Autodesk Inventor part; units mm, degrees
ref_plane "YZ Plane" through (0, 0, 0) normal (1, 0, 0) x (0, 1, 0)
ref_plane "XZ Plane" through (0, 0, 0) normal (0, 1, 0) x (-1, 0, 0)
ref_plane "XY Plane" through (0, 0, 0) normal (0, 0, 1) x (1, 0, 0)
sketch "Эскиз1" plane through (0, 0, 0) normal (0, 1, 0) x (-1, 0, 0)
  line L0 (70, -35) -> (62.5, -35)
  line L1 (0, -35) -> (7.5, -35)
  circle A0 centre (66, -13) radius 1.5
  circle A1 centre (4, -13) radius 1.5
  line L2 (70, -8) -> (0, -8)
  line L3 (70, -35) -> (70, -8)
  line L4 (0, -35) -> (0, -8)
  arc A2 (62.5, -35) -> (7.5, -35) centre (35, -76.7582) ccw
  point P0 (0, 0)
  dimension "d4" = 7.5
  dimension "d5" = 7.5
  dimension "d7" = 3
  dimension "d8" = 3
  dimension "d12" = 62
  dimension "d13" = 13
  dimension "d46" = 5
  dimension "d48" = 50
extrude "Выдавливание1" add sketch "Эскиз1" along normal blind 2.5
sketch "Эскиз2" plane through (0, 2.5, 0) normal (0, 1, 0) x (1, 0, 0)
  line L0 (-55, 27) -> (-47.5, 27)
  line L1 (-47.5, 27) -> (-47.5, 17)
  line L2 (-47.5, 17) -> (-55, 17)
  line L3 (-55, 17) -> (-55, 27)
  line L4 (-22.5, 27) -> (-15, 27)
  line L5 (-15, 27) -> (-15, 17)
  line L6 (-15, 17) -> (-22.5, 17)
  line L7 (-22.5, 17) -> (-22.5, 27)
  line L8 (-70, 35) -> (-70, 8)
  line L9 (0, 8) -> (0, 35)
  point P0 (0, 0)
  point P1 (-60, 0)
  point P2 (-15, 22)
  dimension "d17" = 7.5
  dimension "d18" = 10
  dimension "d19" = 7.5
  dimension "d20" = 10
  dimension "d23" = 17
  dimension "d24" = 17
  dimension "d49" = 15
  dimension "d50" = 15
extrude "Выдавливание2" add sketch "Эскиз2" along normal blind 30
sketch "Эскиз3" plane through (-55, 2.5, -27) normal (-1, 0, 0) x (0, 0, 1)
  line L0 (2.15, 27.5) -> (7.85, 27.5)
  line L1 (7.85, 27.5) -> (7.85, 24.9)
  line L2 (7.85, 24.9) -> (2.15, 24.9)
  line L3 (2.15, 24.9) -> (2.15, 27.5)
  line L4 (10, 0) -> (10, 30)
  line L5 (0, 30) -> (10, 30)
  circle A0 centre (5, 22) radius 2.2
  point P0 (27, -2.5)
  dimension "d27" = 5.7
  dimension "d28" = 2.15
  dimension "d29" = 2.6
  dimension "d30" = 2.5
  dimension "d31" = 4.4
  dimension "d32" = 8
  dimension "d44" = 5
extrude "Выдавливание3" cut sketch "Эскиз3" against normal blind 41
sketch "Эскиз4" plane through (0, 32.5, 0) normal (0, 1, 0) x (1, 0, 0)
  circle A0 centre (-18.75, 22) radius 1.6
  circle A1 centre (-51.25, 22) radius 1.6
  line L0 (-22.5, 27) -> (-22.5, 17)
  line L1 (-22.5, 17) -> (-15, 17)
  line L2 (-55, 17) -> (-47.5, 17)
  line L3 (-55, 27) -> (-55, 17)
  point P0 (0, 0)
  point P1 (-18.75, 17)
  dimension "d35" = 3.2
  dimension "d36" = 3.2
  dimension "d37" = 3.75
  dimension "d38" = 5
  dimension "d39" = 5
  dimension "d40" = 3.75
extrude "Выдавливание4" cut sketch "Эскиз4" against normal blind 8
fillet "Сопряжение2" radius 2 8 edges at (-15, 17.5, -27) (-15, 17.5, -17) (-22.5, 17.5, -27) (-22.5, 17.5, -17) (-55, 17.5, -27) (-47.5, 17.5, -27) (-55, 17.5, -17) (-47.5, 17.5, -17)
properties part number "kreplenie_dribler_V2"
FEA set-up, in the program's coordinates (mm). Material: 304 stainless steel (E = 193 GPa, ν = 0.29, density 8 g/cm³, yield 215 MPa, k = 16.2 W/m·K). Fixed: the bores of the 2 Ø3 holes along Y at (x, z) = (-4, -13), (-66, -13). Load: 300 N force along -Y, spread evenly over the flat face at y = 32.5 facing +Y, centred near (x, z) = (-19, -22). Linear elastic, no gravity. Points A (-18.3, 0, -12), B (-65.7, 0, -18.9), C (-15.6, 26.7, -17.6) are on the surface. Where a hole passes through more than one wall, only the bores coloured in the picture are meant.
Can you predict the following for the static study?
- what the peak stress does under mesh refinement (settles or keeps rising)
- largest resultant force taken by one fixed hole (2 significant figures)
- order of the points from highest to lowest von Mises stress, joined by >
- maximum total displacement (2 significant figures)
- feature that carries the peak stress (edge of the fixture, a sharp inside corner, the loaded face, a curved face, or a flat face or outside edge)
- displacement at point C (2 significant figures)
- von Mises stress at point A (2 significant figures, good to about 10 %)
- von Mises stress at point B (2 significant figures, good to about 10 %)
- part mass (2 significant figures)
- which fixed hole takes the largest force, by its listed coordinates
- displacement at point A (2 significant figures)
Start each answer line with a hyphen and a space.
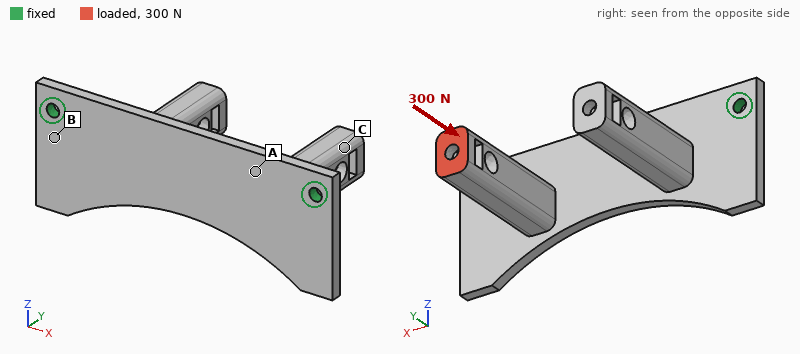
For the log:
- keeps rising
- 250 N
- B > A > C
- 0.14 mm
- edge of the fixture
- 0.10 mm
- 26 MPa
- 48 MPa
- 62 g
- (-4, -13)
- 0.024 mm
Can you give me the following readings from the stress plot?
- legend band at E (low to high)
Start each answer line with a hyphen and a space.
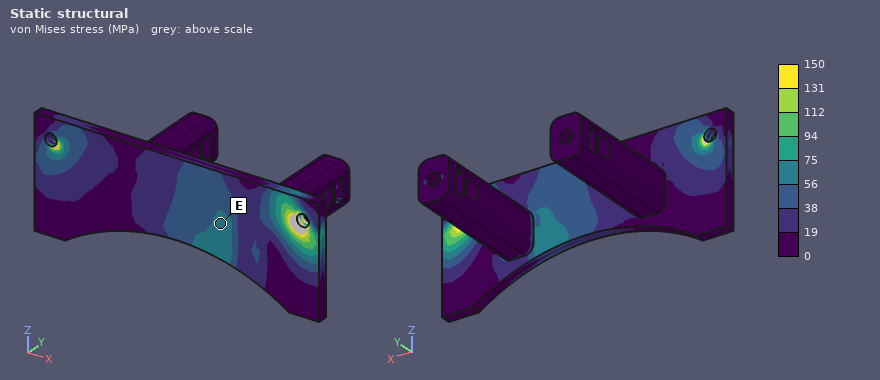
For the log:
- 56 to 75 MPa
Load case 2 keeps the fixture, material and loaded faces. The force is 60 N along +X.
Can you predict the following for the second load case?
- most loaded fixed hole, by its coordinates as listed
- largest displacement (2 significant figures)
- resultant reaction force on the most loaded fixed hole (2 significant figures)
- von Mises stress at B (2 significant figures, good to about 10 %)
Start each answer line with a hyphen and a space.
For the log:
- (-4, -13)
- 69 µm
- 48 N
- 19 MPa
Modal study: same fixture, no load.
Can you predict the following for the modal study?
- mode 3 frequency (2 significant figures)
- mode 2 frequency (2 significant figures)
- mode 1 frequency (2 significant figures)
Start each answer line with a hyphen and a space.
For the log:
- 2100 Hz
- 1700 Hz
- 1200 Hz
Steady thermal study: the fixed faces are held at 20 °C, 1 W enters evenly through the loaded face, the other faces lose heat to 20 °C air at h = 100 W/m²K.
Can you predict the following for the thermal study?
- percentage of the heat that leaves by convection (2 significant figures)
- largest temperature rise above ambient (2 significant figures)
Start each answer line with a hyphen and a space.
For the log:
- 95 %
- 18 K
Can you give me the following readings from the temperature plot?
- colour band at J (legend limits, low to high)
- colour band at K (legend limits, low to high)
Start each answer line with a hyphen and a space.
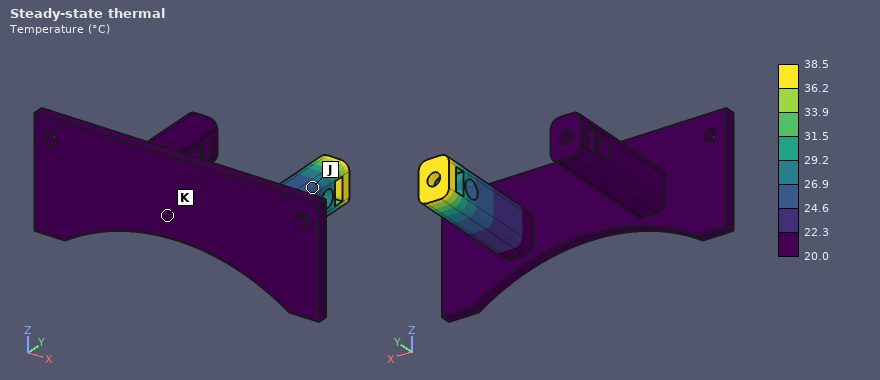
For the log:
- 24.6 to 26.9 °C
- 20.0 to 22.3 °C
